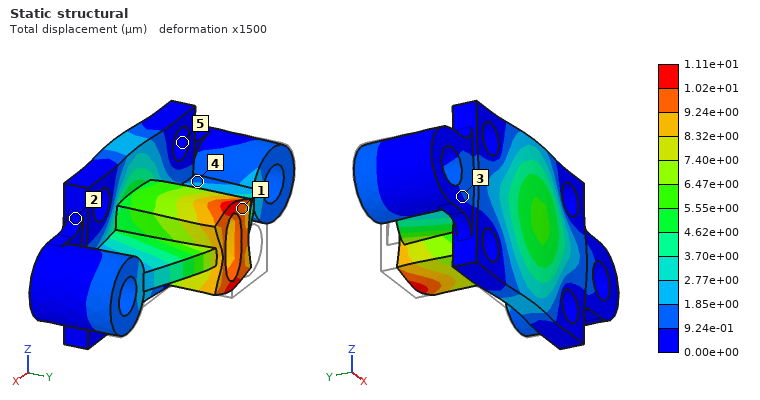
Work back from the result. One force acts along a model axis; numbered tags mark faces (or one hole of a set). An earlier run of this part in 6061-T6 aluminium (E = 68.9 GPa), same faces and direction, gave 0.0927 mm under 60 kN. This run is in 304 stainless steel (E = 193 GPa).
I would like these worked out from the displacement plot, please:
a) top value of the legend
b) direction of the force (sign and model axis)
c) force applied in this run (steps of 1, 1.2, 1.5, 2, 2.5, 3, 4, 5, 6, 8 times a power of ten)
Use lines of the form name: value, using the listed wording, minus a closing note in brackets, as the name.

top value of the legend: 1.11e+01 µm
direction of the force: -Y
force applied in this run: 20 kN
